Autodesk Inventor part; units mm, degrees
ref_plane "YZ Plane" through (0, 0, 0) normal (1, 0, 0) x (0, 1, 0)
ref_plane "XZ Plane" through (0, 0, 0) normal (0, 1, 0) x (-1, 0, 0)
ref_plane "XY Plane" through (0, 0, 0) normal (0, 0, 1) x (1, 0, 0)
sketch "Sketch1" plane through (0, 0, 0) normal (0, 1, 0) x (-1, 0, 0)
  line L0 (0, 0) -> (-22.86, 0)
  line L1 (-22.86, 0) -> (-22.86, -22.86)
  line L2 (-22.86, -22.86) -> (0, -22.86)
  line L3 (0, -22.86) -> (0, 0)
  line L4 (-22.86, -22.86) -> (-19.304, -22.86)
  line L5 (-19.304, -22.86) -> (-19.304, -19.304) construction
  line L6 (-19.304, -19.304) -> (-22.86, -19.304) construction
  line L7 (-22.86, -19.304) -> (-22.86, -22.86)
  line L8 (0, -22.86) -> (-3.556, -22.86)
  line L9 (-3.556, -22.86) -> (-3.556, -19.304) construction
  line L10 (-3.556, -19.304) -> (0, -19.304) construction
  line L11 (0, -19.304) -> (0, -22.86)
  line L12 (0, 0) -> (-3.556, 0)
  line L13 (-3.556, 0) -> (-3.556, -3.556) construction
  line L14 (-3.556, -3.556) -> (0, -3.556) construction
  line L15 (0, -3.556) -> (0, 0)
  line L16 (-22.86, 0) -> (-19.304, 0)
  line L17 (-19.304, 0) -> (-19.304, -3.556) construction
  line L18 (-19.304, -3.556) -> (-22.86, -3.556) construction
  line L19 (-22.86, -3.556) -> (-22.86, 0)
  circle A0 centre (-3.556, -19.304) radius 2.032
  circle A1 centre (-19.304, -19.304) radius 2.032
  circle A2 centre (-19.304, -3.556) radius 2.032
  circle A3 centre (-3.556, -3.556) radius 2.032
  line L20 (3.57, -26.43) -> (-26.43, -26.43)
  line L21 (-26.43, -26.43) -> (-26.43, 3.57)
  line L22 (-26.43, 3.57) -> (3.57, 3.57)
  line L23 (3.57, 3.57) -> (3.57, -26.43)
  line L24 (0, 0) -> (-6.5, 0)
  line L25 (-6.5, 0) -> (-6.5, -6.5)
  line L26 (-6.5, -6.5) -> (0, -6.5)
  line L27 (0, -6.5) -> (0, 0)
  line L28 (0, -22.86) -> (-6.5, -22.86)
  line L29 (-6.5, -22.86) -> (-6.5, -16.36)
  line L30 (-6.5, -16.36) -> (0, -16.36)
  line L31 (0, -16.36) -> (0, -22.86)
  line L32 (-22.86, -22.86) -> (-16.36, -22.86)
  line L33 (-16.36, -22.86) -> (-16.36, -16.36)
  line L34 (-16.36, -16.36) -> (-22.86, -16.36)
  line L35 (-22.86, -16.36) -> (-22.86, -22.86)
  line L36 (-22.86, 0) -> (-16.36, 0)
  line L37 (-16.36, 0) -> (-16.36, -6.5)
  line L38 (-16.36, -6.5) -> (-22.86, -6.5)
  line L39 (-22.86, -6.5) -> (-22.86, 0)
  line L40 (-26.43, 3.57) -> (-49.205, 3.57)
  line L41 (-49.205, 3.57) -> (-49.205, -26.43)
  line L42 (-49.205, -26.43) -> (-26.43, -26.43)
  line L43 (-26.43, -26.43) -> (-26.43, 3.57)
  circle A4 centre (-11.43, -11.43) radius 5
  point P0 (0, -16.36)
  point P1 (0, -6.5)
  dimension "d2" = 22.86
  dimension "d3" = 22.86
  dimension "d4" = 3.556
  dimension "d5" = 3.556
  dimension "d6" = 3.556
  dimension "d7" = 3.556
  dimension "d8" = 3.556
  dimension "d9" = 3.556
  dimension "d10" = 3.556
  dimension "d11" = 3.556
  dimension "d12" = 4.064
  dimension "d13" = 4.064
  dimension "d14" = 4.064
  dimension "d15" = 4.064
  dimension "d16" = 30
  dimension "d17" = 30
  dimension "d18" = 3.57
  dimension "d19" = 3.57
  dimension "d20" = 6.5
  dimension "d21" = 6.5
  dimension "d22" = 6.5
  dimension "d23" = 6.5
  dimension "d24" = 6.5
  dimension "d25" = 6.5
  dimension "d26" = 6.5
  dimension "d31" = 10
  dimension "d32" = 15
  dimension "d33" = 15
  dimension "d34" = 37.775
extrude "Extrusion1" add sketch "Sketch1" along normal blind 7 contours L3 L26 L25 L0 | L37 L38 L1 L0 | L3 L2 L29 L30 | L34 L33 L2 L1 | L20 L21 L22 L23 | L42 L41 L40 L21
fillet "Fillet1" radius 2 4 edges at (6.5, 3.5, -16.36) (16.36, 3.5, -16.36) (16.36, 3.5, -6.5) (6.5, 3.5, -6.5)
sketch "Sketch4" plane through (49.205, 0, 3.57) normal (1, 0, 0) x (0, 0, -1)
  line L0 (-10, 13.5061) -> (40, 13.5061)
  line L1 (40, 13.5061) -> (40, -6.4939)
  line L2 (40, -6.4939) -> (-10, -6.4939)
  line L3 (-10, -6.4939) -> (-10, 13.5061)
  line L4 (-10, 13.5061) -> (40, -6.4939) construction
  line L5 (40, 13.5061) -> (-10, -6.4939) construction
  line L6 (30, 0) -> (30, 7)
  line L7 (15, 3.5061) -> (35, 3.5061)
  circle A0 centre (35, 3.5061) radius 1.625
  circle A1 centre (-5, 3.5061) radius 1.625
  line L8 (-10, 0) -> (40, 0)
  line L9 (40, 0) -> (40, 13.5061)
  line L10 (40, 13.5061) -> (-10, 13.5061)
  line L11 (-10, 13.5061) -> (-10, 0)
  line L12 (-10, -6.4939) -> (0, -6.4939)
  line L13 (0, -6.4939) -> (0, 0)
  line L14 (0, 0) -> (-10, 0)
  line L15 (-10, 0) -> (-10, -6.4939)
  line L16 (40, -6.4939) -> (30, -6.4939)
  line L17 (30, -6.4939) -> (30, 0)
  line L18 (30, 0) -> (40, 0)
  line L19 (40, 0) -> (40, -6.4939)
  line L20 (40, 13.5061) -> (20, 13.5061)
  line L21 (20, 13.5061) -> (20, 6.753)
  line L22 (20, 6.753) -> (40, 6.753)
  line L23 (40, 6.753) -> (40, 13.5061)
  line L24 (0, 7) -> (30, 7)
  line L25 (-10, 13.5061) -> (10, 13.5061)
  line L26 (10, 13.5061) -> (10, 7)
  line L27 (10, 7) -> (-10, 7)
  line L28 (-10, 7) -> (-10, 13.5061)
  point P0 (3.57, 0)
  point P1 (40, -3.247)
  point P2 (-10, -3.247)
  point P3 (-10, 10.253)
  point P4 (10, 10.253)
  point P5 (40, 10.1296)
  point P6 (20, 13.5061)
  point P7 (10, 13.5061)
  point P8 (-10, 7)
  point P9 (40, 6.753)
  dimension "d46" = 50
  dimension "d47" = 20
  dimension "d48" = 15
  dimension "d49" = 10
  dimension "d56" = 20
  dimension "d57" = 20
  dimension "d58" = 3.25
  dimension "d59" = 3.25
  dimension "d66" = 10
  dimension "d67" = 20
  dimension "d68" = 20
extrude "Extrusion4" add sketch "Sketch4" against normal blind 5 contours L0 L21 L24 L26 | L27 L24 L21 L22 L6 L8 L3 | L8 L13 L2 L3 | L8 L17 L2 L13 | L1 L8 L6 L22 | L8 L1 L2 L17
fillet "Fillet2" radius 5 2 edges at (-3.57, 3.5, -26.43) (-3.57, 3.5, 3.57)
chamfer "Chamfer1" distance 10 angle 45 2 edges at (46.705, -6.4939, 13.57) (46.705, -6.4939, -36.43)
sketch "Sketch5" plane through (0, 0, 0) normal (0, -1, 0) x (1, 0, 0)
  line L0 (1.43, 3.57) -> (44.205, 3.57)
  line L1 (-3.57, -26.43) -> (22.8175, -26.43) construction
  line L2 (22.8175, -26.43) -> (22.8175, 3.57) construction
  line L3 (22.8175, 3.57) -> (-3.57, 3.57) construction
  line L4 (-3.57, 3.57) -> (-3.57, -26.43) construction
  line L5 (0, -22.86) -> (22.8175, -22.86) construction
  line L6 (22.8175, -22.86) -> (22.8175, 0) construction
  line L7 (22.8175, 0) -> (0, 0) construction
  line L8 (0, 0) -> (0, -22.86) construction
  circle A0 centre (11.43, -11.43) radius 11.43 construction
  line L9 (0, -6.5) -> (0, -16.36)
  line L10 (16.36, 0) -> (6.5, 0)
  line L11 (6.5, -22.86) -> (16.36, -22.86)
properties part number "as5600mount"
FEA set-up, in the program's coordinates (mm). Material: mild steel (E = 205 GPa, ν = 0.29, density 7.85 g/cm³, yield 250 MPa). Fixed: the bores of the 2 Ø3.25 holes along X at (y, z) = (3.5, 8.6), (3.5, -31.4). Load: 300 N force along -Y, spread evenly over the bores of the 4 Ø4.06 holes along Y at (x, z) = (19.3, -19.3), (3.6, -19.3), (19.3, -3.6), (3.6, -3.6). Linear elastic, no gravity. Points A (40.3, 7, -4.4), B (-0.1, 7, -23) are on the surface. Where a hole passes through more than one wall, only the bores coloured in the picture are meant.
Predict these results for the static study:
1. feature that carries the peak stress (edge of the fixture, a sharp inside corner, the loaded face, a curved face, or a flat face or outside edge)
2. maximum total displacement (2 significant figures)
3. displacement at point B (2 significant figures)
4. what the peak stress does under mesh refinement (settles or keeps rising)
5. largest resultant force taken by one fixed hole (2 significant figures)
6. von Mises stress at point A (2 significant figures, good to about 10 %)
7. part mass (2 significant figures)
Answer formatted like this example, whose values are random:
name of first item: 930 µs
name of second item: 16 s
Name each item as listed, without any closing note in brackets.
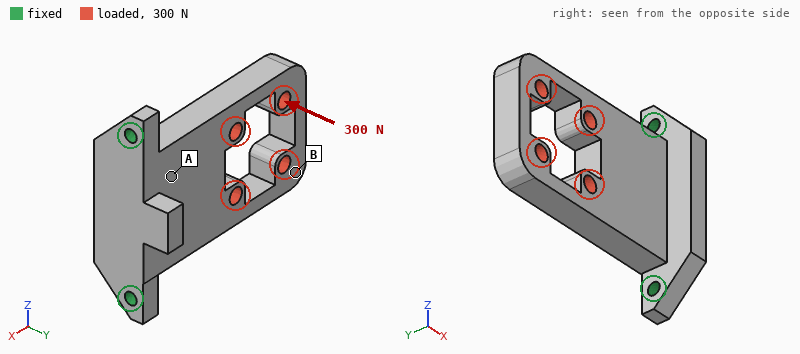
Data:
feature that carries the peak stress: edge of the fixture
maximum total displacement: 0.13 mm
displacement at point B: 0.11 mm
what the peak stress does under mesh refinement: keeps rising
largest resultant force taken by one fixed hole: 190 N
von Mises stress at point A: 31 MPa
part mass: 80 g
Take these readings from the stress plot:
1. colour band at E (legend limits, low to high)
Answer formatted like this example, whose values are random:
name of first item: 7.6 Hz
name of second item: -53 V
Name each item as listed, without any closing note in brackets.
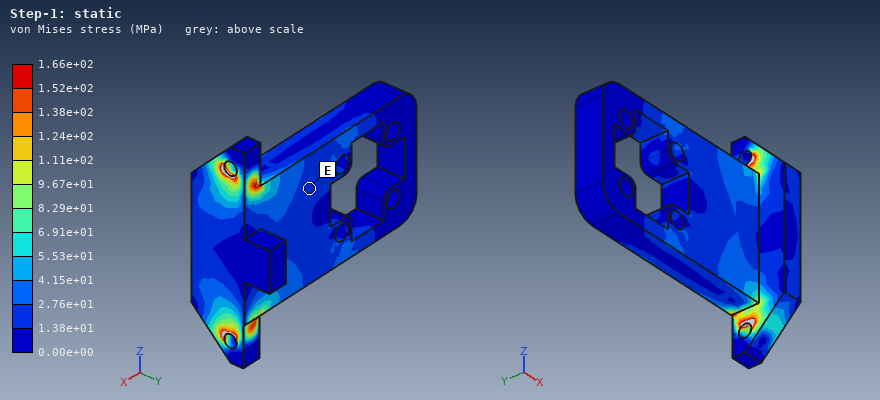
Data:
colour band at E: 1.38e+01 to 2.76e+01 MPa
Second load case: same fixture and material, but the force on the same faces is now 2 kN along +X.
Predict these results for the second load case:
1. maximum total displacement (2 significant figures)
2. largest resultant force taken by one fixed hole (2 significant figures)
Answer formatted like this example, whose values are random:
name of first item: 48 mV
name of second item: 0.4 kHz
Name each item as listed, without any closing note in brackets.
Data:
maximum total displacement: 18 µm
largest resultant force taken by one fixed hole: 1.1 kN
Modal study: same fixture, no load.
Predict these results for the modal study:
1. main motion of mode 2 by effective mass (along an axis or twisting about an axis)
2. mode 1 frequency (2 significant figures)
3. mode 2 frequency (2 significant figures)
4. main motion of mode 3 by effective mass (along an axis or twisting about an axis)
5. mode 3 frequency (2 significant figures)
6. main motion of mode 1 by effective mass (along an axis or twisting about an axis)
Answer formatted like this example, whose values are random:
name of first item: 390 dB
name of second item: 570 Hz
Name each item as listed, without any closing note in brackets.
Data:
main motion of mode 2 by effective mass: along Z
mode 1 frequency: 1700 Hz
mode 2 frequency: 5100 Hz
main motion of mode 3 by effective mass: twisting about X
mode 3 frequency: 6100 Hz
main motion of mode 1 by effective mass: along Y
